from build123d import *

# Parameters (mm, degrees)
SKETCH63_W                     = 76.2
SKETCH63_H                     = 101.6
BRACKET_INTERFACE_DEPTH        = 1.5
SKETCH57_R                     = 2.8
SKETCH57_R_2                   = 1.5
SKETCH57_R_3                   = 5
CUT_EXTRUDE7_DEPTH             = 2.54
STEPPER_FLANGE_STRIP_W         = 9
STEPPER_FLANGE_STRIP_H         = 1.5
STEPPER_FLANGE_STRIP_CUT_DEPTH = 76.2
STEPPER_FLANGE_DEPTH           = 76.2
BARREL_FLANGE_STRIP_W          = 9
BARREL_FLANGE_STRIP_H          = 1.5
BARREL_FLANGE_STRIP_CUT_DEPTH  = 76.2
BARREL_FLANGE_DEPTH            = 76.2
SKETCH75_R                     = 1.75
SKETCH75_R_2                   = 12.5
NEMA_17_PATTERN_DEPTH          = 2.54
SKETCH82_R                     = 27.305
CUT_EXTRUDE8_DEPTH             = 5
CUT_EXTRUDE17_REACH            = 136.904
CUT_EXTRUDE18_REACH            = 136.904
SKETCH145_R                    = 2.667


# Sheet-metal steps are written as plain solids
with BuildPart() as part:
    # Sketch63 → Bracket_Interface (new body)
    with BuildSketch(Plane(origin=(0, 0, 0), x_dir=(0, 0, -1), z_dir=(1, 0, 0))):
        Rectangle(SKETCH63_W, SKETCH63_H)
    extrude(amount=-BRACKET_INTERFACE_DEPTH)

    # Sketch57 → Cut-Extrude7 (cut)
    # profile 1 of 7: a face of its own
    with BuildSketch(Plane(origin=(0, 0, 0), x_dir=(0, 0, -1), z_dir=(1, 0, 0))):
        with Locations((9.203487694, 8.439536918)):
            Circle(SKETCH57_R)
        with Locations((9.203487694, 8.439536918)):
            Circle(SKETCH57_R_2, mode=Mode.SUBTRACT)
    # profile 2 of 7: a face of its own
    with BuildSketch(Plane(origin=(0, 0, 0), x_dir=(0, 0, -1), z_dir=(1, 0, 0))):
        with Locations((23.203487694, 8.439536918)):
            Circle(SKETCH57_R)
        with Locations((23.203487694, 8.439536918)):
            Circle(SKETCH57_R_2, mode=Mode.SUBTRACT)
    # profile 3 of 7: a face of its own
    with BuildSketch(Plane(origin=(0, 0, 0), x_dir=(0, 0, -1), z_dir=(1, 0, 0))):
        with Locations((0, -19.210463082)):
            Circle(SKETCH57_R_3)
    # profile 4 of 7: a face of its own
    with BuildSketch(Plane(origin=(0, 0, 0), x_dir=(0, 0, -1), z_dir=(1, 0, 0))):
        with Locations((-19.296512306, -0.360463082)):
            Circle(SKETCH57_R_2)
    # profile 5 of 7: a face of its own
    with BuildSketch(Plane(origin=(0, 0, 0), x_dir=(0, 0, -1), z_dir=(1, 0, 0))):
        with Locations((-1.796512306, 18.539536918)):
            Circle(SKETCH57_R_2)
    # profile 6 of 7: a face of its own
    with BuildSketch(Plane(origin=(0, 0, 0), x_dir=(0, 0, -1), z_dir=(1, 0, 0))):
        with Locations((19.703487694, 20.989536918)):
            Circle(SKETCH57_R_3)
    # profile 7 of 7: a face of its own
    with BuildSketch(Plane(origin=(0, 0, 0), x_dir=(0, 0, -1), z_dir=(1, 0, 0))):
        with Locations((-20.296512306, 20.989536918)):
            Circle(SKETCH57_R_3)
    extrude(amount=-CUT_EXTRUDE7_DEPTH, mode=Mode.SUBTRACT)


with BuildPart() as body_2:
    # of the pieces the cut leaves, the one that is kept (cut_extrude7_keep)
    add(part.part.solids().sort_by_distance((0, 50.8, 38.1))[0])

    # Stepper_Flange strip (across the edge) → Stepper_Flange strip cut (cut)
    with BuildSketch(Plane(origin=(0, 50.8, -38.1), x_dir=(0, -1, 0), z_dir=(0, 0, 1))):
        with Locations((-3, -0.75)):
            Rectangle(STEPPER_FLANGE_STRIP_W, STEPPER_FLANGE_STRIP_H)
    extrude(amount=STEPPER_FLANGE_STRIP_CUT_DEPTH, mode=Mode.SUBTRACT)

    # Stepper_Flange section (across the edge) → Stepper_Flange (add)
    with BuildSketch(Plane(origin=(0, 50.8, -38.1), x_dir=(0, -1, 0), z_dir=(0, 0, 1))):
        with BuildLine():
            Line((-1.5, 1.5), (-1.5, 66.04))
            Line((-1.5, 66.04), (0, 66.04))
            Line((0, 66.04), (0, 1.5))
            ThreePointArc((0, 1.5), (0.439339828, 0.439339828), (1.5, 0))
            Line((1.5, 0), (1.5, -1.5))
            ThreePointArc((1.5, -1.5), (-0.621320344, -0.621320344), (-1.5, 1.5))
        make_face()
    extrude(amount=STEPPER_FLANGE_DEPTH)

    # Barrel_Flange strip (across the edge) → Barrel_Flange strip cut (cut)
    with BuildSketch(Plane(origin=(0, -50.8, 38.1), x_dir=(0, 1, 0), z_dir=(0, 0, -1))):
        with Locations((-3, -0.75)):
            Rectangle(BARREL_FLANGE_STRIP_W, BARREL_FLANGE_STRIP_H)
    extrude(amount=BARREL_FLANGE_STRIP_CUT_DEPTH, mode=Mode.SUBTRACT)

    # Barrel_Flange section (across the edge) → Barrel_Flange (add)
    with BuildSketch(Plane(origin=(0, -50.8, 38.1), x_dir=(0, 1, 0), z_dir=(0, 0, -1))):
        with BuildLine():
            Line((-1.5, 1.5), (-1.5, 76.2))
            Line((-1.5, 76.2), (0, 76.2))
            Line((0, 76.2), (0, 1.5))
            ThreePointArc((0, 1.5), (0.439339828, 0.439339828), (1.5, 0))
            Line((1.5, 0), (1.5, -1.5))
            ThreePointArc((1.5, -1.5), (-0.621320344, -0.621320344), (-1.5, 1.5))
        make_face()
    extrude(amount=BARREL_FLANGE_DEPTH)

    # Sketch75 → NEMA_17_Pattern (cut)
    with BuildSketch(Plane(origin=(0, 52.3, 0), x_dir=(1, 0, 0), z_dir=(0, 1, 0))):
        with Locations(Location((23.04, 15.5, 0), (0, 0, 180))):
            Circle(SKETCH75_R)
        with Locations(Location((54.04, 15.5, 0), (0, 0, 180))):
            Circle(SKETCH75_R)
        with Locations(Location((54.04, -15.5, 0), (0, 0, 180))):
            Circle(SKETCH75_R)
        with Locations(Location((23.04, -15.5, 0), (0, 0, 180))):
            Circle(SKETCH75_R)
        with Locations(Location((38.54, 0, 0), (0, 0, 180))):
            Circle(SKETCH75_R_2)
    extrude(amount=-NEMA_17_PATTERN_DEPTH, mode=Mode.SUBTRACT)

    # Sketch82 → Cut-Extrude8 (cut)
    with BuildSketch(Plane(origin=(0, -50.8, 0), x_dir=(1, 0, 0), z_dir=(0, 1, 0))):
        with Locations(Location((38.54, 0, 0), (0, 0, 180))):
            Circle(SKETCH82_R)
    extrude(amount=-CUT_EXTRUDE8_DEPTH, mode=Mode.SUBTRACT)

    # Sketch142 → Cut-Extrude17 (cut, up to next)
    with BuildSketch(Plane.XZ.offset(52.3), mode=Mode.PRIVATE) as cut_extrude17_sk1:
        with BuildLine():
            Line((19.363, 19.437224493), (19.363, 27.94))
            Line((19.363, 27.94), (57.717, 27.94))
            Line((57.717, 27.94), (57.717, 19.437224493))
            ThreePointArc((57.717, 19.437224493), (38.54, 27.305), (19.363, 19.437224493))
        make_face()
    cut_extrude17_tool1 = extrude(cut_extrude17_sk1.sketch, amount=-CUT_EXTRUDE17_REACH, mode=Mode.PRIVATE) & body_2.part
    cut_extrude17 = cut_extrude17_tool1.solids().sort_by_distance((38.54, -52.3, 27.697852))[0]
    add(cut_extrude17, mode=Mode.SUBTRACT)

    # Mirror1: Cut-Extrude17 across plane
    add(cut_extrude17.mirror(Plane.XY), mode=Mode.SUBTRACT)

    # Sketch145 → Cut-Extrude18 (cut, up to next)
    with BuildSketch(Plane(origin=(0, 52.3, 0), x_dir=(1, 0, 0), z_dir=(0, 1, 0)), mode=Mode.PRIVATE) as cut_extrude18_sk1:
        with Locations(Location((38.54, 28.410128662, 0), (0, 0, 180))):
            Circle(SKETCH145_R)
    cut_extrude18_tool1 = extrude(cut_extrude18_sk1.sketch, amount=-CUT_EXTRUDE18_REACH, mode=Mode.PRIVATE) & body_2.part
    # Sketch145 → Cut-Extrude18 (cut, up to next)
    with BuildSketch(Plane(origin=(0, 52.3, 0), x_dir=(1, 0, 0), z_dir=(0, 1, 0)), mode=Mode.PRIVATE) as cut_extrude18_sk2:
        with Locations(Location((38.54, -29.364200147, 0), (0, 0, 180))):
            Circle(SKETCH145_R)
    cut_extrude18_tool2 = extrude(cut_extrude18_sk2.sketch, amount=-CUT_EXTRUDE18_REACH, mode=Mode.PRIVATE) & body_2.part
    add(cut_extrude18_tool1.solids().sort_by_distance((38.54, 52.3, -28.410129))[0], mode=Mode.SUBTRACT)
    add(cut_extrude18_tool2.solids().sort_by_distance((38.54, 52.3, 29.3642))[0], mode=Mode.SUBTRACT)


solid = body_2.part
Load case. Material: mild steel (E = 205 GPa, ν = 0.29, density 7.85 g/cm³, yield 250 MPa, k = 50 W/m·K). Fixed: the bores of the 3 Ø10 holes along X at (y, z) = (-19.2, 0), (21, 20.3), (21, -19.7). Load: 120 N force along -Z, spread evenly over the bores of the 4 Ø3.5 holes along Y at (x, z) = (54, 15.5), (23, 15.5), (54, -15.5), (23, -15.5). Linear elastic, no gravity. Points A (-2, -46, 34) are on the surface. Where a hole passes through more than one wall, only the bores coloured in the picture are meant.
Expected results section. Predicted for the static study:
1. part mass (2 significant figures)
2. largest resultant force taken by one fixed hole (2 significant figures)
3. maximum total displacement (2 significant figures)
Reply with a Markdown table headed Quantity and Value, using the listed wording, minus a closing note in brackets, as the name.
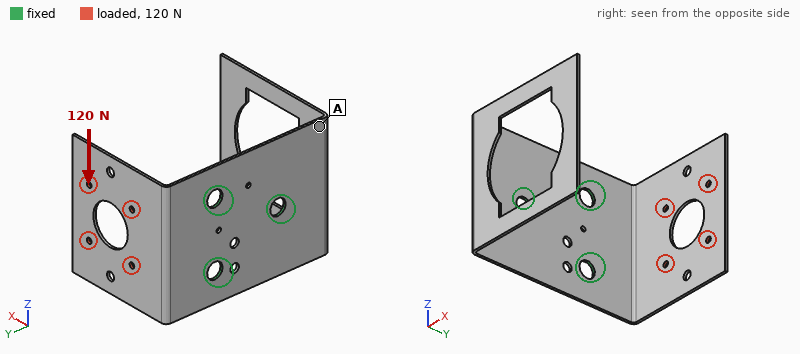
| Quantity | Value |
|---|---|
| part mass | 180 g |
| largest resultant force taken by one fixed hole | 130 N |
| maximum total displacement | 0.51 mm |
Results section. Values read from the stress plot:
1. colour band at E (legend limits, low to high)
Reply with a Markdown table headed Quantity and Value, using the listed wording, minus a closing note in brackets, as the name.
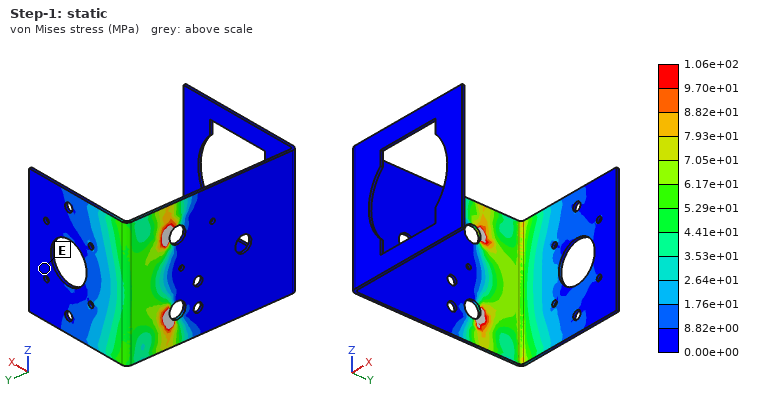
| Quantity | Value |
|---|---|
| colour band at E | 0.00e+00 to 8.82e+00 MPa |
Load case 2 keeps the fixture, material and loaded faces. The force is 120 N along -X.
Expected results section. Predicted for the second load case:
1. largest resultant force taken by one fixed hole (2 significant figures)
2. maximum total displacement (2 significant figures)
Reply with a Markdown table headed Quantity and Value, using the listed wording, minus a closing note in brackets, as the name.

| Quantity | Value |
|---|---|
| largest resultant force taken by one fixed hole | 63 N |
| maximum total displacement | 0.70 mm |
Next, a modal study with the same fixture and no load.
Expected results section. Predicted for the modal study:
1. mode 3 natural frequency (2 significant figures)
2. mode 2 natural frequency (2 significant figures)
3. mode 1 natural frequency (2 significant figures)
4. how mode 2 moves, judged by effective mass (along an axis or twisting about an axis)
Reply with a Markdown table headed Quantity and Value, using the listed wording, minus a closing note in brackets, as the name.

| Quantity | Value |
|---|---|
| mode 3 natural frequency | 230 Hz |
| mode 2 natural frequency | 180 Hz |
| mode 1 natural frequency | 130 Hz |
| how mode 2 moves, judged by effective mass | along Y |
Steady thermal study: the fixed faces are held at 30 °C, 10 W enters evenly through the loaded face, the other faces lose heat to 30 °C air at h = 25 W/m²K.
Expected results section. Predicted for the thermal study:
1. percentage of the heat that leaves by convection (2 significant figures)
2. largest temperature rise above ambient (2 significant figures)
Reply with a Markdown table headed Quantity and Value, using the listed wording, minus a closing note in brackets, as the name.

| Quantity | Value |
|---|---|
| percentage of the heat that leaves by convection | 78 % |
| largest temperature rise above ambient | 49 K |
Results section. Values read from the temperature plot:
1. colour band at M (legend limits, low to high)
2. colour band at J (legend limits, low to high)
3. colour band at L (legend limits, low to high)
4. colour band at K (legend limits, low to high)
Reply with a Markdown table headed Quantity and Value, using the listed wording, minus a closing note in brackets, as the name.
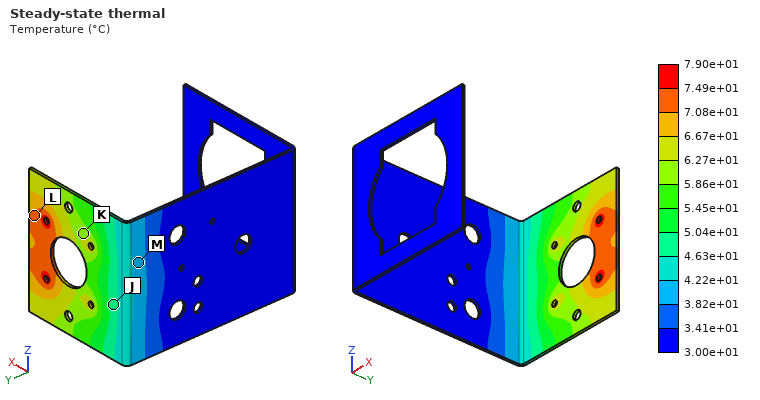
| Quantity | Value |
|---|---|
| colour band at M | 3.82e+01 to 4.22e+01 °C |
| colour band at J | 4.63e+01 to 5.04e+01 °C |
| colour band at L | 7.08e+01 to 7.49e+01 °C |
| colour band at K | 5.86e+01 to 6.27e+01 °C |
